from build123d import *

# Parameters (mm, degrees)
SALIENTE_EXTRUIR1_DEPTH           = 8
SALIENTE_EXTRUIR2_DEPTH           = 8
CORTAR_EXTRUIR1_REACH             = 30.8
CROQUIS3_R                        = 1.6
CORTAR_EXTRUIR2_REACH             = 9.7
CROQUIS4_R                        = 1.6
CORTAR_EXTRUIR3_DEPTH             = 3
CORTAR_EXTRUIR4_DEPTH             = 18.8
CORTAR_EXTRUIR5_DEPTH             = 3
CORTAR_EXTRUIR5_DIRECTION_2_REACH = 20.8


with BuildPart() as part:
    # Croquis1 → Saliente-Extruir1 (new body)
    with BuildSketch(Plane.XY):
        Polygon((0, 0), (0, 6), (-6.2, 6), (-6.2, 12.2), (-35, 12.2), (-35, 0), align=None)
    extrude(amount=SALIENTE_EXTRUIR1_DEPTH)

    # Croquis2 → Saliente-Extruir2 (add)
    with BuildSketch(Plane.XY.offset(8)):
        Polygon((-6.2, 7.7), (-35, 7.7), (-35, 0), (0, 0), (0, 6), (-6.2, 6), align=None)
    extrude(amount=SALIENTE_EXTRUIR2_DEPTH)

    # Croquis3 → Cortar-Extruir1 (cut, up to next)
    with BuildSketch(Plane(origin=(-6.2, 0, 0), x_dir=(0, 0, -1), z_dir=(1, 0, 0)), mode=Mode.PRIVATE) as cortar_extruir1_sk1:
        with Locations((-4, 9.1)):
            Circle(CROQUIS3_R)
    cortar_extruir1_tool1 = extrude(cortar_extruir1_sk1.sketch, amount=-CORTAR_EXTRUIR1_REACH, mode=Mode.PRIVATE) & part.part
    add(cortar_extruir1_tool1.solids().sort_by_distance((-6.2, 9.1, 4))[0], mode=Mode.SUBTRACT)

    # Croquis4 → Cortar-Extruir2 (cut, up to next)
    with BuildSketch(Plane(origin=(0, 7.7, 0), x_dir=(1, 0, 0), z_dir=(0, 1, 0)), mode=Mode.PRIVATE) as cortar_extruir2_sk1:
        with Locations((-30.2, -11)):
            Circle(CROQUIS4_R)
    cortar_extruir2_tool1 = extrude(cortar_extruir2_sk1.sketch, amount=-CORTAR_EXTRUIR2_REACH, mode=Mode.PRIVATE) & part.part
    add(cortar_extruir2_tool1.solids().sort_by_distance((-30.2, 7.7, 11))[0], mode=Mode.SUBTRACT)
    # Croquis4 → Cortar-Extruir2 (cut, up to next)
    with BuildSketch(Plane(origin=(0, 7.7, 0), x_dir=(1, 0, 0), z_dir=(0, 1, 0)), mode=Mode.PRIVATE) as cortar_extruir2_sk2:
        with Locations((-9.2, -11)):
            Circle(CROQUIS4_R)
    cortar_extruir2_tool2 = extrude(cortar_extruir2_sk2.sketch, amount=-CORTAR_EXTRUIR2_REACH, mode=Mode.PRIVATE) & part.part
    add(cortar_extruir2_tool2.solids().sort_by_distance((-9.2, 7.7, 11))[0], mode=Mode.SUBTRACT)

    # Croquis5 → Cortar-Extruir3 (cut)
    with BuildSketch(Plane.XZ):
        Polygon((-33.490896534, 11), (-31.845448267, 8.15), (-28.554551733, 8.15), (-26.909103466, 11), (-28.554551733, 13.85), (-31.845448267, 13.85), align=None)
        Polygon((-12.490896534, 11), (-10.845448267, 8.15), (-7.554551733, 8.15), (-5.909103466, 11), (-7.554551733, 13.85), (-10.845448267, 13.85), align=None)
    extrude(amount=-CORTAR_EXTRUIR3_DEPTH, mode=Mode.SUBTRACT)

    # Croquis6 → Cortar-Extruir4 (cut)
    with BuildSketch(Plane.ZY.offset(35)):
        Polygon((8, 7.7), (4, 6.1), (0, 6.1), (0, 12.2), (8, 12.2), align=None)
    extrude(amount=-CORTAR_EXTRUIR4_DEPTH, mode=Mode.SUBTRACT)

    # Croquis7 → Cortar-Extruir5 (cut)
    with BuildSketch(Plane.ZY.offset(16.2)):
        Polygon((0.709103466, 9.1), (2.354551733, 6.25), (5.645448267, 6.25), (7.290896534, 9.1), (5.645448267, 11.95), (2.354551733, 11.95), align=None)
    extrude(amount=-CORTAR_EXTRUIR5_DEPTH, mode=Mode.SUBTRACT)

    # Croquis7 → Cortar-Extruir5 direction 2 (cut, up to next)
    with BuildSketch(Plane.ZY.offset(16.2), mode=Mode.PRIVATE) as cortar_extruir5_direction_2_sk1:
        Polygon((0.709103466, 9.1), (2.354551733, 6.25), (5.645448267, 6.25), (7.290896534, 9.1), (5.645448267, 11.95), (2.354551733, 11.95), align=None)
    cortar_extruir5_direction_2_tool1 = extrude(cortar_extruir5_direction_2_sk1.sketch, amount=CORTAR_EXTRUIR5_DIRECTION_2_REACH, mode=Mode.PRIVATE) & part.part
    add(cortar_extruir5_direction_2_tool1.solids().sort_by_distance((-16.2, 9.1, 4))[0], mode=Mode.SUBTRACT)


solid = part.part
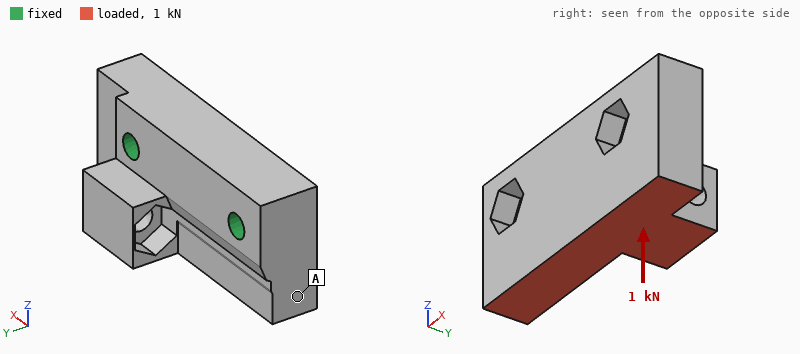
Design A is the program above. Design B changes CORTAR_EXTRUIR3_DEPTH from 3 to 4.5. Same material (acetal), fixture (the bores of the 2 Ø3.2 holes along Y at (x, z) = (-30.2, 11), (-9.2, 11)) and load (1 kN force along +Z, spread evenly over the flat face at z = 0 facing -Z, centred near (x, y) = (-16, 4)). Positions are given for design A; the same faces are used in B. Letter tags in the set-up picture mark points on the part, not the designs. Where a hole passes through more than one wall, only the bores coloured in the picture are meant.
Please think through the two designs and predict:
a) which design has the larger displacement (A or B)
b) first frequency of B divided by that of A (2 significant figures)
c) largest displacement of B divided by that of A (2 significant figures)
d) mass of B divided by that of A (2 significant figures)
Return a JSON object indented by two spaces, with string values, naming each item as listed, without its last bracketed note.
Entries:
{
  "which design has the larger displacement": "B",
  "first frequency of B divided by that of A": "0.73",
  "largest displacement of B divided by that of A": "1.6",
  "mass of B divided by that of A": "0.98"
}
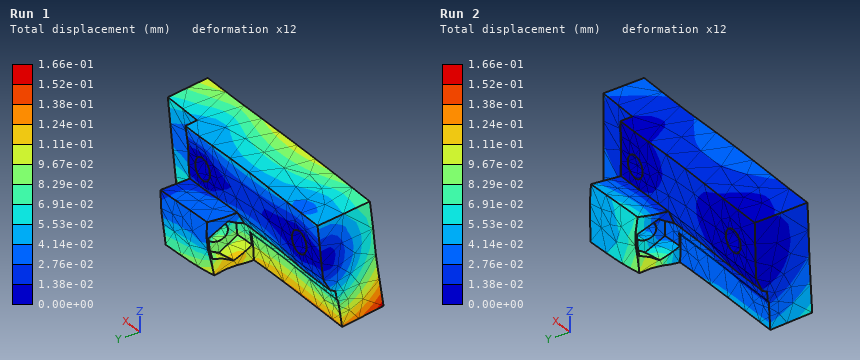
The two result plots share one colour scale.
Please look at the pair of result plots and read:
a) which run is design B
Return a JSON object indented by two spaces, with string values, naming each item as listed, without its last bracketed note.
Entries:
{
  "which run is design B": "Run 1"
}
